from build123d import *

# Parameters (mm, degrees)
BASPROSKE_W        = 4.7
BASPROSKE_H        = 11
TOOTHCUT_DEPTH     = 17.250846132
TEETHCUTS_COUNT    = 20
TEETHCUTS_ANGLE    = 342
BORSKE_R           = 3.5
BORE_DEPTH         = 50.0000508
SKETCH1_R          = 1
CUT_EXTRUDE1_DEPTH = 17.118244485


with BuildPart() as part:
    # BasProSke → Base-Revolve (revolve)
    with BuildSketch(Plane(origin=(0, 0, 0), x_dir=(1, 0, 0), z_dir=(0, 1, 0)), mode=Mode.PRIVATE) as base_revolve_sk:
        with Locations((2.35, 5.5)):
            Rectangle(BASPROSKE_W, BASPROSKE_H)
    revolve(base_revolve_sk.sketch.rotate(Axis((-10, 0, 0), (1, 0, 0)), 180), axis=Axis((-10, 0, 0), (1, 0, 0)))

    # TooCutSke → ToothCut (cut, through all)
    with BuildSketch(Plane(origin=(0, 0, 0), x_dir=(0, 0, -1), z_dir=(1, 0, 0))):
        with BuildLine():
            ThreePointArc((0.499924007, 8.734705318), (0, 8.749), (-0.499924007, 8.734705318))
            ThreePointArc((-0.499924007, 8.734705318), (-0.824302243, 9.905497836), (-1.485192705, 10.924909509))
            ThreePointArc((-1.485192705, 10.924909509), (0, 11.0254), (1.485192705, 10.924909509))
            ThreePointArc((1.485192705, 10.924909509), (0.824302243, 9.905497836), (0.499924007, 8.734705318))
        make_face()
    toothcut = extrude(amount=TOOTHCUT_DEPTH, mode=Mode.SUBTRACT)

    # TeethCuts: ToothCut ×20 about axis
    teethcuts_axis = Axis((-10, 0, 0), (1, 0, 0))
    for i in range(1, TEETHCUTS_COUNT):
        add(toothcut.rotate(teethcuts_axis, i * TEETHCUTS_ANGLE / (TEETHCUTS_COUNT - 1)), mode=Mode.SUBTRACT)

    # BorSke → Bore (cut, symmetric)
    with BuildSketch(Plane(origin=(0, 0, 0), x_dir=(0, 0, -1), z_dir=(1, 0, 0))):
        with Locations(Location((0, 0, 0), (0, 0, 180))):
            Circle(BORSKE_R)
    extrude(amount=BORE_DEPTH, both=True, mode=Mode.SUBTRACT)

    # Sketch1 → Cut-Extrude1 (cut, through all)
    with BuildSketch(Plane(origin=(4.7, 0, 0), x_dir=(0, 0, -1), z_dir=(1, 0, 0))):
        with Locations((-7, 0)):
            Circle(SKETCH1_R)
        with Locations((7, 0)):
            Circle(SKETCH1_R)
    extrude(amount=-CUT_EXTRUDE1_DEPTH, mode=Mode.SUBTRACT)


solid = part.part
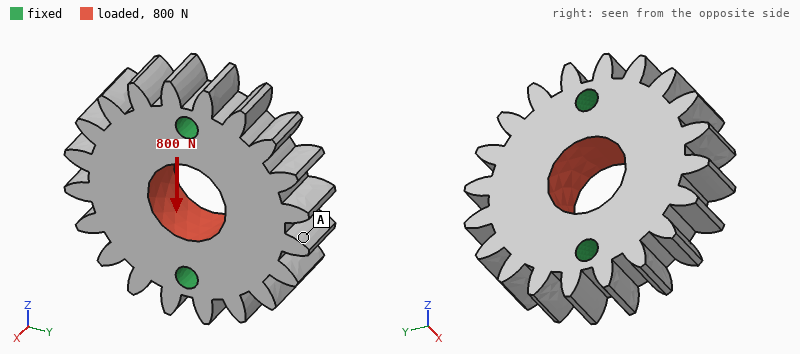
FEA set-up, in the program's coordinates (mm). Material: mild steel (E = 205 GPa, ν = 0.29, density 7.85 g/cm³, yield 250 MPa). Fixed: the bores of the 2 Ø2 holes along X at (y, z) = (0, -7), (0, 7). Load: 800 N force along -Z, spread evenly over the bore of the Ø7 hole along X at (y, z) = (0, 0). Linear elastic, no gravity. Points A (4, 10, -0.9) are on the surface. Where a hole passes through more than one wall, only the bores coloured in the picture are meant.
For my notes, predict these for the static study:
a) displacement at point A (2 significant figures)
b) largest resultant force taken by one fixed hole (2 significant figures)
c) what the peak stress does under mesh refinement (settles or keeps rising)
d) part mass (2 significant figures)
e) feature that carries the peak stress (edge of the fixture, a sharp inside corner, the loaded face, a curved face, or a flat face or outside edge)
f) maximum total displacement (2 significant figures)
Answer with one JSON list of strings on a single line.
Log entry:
["0.26 µm", "400 N", "keeps rising", "9.5 g", "edge of the fixture", "0.53 µm"]
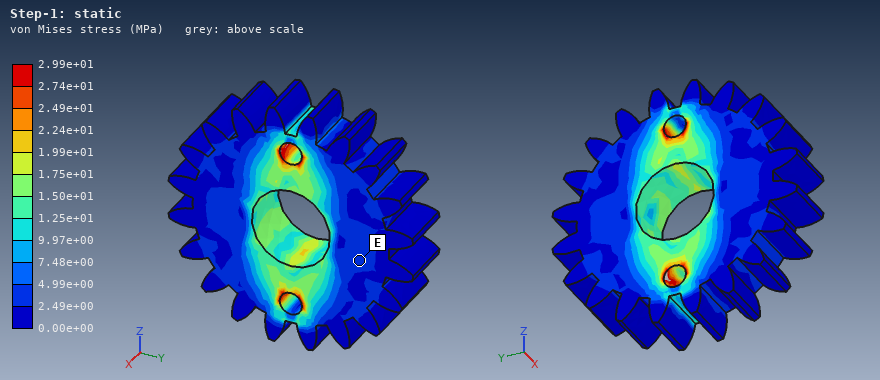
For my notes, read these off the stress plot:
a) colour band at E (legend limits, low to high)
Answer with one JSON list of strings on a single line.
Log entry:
["2.49e+00 to 4.99e+00 MPa"]
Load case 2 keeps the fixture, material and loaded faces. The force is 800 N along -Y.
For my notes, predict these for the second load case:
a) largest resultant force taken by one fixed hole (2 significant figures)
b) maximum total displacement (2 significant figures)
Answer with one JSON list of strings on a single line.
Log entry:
["400 N", "0.58 µm"]
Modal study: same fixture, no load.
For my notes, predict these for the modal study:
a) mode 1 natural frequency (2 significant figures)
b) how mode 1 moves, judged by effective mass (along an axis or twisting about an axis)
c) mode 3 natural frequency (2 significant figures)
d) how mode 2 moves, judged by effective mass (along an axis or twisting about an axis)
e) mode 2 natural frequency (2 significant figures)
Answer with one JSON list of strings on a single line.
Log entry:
["30 kHz", "twisting about Z", "63 kHz", "along X", "34 kHz"]
